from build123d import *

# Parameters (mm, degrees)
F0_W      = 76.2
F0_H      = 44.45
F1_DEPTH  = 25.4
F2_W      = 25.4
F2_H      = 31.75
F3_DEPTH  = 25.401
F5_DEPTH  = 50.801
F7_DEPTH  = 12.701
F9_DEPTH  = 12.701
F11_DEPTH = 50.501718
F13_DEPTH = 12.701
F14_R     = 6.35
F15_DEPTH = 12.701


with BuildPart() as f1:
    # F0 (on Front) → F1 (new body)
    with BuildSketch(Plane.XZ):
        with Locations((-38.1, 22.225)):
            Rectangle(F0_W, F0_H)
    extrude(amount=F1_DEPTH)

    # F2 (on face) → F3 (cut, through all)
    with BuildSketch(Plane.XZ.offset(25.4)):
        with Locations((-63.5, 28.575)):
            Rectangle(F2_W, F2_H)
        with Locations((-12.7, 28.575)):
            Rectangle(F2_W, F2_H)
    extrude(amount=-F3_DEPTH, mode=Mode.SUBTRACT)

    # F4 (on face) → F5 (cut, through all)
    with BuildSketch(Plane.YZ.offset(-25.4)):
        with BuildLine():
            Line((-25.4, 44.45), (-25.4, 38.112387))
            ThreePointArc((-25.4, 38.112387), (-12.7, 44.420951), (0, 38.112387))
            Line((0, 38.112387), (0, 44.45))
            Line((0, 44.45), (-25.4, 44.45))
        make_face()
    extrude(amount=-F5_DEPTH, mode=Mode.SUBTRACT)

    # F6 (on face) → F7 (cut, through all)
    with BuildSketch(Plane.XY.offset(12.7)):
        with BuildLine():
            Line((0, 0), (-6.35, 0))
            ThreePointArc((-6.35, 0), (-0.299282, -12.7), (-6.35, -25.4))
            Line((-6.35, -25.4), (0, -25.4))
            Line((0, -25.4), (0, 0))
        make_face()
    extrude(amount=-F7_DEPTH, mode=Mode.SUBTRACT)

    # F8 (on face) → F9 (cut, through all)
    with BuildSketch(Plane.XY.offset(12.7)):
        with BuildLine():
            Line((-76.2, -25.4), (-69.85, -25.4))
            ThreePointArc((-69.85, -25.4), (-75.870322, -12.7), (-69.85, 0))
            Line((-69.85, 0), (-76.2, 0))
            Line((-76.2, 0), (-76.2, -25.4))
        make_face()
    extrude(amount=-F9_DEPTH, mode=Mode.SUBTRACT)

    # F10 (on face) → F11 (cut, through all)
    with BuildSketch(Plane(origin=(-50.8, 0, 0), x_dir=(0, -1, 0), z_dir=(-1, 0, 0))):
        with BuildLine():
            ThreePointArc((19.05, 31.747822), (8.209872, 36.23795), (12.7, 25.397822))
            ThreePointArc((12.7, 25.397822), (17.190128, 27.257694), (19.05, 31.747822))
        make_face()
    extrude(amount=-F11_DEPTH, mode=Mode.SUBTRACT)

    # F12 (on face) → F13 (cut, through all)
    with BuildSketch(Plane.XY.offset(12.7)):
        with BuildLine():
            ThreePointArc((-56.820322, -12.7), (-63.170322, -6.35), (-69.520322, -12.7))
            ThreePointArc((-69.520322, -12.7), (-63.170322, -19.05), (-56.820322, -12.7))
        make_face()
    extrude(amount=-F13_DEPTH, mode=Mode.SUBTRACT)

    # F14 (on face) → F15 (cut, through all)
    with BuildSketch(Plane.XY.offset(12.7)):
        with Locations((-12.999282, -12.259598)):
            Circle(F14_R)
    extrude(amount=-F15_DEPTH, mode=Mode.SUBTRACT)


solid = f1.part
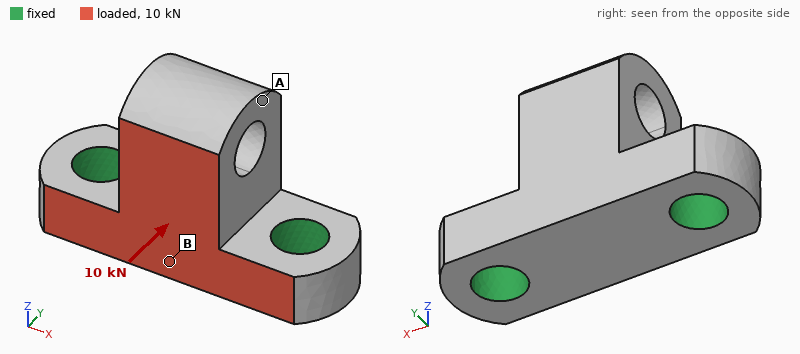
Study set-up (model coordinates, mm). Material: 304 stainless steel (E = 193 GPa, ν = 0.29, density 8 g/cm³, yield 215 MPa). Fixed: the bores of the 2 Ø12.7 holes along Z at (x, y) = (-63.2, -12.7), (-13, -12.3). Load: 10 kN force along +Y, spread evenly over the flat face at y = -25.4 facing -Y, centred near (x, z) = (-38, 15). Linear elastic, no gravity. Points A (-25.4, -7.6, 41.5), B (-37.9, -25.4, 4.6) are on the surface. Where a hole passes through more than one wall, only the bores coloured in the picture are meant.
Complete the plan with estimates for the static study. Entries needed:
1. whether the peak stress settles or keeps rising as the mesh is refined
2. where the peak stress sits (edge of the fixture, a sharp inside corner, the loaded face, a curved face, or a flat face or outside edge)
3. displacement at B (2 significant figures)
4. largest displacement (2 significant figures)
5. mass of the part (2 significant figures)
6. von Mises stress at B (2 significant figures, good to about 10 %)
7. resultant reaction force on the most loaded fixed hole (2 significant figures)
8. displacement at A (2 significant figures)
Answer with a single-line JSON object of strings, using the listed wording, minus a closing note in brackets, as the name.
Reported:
{"whether the peak stress settles or keeps rising as the mesh is refined": "keeps rising", "where the peak stress sits": "edge of the fixture", "displacement at B": "6.5 µm", "largest displacement": "26 µm", "mass of the part": "290 g", "von Mises stress at B": "22 MPa", "resultant reaction force on the most loaded fixed hole": "5.0 kN", "displacement at A": "24 µm"}
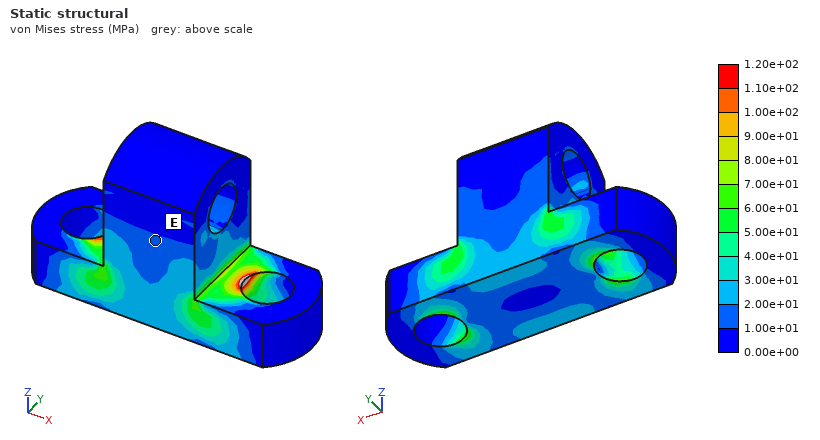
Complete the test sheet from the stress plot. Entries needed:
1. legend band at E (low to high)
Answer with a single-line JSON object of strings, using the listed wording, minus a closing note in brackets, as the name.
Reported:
{"legend band at E": "1.00e+01 to 2.00e+01 MPa"}
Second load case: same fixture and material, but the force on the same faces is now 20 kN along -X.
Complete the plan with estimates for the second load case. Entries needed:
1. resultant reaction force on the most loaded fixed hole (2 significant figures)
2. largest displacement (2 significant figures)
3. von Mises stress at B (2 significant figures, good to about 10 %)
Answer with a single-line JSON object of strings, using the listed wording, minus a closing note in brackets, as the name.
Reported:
{"resultant reaction force on the most loaded fixed hole": "12 kN", "largest displacement": "25 µm", "von Mises stress at B": "24 MPa"}
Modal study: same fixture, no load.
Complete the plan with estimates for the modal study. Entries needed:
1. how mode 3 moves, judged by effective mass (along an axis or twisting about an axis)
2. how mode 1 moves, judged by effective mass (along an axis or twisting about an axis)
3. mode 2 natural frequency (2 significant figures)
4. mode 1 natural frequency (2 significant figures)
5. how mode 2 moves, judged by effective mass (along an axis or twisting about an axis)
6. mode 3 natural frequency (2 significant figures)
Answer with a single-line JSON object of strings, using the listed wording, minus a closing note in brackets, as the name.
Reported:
{"how mode 3 moves, judged by effective mass": "along Z", "how mode 1 moves, judged by effective mass": "along Y", "mode 2 natural frequency": "11 kHz", "mode 1 natural frequency": "6600 Hz", "how mode 2 moves, judged by effective mass": "along X", "mode 3 natural frequency": "17 kHz"}
